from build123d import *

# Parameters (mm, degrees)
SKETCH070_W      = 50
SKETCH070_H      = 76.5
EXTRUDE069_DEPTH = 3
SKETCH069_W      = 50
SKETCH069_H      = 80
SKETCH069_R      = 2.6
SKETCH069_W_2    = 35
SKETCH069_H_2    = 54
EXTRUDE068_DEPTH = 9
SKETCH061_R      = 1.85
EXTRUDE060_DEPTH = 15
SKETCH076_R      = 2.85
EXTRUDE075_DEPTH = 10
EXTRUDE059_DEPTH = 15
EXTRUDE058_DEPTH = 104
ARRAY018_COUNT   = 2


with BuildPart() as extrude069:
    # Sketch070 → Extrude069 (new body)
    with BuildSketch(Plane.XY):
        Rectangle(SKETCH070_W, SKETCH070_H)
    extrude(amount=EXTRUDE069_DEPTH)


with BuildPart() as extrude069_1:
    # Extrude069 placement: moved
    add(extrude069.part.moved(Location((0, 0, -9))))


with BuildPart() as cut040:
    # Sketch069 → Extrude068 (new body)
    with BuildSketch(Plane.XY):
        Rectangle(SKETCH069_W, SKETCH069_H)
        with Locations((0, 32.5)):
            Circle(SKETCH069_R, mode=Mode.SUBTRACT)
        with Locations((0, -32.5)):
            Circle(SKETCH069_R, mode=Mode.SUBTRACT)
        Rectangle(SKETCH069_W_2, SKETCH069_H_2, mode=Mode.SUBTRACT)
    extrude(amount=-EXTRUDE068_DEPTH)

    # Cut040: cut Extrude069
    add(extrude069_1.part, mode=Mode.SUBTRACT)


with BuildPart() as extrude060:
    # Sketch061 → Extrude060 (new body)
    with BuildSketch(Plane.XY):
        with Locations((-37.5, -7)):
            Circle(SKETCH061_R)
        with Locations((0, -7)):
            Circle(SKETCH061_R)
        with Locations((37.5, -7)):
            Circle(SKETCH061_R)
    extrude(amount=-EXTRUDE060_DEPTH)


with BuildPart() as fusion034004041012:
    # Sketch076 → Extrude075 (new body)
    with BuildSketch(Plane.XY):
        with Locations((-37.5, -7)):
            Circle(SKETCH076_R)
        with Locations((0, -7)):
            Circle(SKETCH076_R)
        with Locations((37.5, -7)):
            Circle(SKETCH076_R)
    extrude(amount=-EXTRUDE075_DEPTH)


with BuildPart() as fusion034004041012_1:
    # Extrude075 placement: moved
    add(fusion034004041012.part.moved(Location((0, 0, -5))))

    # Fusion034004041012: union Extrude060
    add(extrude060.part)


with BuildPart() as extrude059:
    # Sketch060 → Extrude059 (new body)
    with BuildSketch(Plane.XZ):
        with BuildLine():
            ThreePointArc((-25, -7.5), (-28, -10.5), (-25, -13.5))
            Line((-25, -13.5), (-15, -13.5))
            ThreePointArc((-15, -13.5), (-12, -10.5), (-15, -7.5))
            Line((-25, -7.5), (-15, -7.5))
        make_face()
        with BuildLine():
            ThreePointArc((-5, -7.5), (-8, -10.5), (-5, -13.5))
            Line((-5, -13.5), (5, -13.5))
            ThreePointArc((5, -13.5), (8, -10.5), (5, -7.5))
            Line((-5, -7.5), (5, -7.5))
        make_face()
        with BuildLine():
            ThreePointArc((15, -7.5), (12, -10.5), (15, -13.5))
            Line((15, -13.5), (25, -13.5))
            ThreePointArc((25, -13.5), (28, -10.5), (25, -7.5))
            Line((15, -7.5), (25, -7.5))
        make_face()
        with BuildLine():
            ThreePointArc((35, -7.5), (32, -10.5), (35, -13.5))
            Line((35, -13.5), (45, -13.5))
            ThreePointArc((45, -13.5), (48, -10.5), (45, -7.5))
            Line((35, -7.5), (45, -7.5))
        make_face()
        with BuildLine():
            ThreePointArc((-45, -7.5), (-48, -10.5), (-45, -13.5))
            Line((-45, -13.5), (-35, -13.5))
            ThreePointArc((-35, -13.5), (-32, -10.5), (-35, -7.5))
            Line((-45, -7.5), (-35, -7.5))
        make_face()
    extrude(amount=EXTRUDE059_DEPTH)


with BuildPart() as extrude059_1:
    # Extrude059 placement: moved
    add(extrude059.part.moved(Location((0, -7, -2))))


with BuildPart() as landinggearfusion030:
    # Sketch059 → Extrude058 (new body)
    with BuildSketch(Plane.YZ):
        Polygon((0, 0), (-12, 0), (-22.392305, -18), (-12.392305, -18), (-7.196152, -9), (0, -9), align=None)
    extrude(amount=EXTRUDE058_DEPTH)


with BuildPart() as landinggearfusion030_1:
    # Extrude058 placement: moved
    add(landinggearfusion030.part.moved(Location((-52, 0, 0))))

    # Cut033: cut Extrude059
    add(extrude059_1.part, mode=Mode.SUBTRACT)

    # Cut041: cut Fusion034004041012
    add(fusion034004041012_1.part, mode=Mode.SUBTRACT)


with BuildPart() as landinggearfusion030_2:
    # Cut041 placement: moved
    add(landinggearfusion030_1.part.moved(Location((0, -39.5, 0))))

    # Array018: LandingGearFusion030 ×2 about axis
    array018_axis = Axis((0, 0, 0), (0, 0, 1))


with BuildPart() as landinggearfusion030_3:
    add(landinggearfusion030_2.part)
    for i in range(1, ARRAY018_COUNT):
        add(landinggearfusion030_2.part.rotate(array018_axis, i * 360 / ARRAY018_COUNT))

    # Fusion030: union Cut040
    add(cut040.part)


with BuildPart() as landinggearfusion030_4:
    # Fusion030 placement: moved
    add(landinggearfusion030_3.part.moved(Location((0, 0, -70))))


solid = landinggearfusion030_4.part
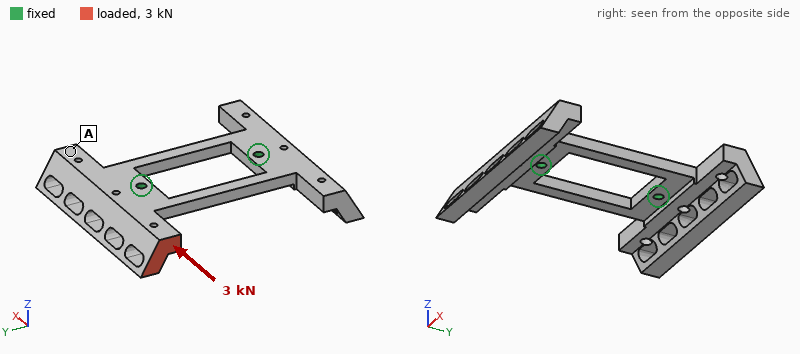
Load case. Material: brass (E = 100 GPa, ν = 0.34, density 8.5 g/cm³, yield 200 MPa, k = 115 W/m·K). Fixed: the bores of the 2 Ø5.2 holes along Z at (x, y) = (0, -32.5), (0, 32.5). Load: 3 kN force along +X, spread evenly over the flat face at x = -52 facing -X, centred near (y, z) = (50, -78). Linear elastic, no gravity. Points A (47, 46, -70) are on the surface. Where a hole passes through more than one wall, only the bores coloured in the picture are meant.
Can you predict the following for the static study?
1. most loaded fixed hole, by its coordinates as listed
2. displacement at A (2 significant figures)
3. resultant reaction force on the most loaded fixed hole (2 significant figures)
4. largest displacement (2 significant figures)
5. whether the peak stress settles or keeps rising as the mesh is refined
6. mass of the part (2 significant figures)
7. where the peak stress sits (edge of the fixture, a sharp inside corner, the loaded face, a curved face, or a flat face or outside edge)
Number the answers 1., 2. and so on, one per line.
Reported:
1. (0, 32.5)
2. 0.11 mm
3. 3.2 kN
4. 0.17 mm
5. keeps rising
6. 410 g
7. edge of the fixture
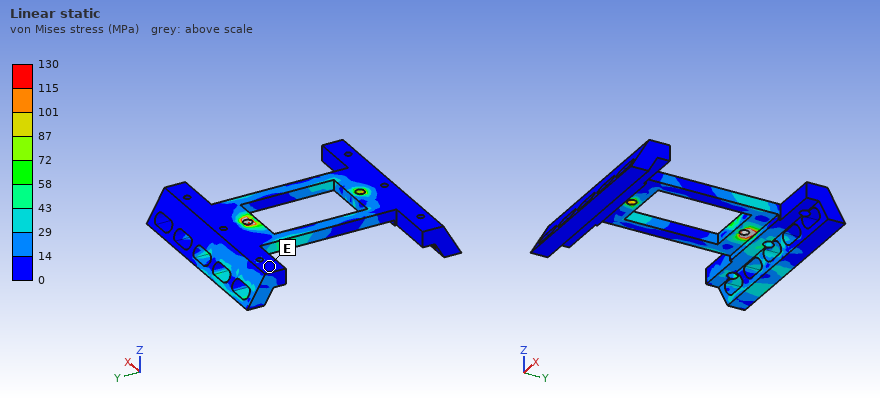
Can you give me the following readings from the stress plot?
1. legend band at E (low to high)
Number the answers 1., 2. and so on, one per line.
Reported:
1. 0 to 14 MPa
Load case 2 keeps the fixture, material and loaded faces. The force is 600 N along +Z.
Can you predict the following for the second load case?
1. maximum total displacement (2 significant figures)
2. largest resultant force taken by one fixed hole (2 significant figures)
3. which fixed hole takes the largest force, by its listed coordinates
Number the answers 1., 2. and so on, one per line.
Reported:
1. 0.38 mm
2. 650 N
3. (0, 32.5)
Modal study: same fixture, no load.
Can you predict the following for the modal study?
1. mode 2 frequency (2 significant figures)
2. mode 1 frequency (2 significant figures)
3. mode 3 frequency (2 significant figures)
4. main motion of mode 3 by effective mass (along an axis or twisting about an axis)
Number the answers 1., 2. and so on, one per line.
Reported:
1. 1100 Hz
2. 1000 Hz
3. 1600 Hz
4. twisting about Z
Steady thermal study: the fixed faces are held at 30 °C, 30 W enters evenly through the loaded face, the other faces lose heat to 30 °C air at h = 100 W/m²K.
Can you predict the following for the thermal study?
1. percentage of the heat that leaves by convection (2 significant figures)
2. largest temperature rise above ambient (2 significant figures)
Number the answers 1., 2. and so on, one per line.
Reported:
1. 53 %
2. 63 K
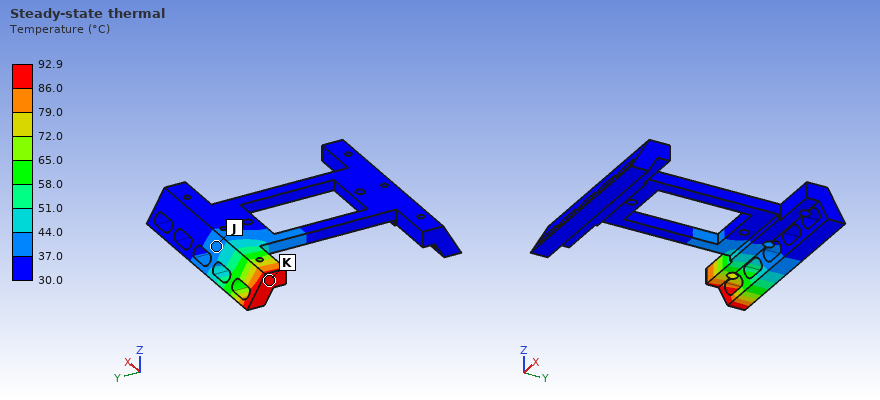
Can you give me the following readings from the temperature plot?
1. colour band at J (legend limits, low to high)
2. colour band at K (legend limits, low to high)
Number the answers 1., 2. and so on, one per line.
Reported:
1. 37.0 to 44.0 °C
2. 86.0 to 92.9 °C
